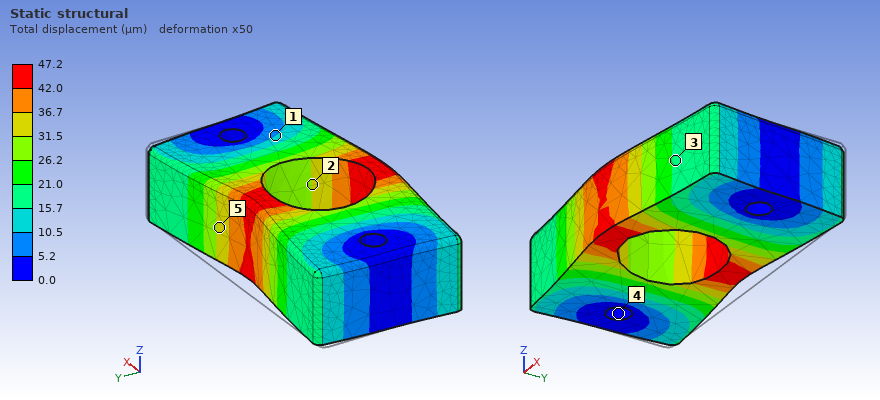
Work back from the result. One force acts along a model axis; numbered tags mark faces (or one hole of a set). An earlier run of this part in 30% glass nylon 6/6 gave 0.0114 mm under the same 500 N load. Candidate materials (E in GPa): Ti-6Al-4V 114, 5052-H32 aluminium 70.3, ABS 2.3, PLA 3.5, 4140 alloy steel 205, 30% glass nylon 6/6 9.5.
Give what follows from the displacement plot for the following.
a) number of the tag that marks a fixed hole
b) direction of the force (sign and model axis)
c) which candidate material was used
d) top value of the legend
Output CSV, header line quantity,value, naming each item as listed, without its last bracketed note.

quantity,value
number of the tag that marks a fixed hole,4
direction of the force,-Y
which candidate material was used,ABS
top value of the legend,47.2 µm
